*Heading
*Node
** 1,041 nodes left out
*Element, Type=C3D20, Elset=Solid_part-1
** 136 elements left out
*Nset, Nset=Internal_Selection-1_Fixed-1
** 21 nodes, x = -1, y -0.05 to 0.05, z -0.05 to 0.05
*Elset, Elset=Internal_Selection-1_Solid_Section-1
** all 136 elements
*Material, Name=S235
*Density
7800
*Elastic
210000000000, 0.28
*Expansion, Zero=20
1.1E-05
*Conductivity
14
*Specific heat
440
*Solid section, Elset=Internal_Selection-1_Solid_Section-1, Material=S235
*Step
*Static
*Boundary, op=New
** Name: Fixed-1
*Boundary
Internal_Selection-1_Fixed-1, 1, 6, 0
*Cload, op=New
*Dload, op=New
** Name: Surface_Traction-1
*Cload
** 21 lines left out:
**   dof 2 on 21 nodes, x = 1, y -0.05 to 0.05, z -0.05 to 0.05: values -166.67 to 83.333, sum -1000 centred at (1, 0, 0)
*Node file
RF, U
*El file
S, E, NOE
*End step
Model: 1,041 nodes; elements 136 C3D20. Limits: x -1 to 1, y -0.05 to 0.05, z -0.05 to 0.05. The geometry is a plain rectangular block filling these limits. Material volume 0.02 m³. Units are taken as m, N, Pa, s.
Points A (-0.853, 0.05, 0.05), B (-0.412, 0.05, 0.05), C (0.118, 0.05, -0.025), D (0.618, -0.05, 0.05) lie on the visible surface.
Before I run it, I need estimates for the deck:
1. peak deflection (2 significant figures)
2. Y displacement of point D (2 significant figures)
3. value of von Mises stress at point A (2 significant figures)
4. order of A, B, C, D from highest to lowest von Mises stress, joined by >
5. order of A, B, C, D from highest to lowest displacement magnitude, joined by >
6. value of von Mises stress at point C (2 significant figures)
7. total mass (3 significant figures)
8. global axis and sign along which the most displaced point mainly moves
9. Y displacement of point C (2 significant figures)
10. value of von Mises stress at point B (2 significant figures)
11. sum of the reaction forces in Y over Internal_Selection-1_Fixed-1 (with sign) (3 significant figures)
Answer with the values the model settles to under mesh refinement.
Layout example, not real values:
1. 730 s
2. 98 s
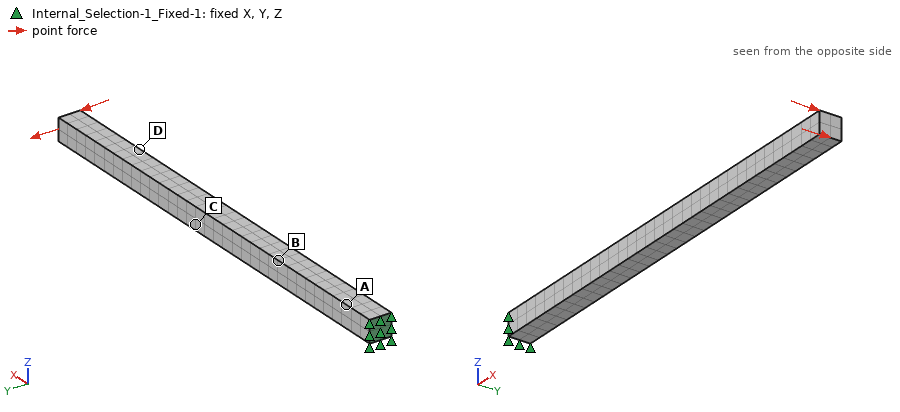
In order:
1. 0.0015 m
2. -0.0011 m
3. 1.1e+07 Pa
4. A > B > C > D
5. D > C > B > A
6. 5.3e+06 Pa
7. 156 kg
8. -Y
9. -5.8e-04 m
10. 8.5e+06 Pa
11. 1000 N
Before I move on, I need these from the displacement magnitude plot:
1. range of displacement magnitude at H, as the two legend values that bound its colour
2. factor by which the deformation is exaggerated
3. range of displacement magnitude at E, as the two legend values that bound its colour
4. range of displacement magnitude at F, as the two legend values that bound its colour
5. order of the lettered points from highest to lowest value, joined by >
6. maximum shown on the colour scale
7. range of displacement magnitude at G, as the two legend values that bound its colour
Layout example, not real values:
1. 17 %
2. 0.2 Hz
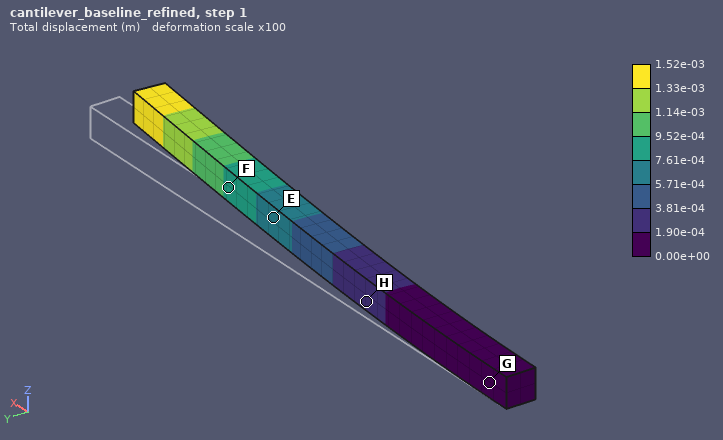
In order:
1. 1.90e-04 to 3.81e-04 m
2. 100
3. 5.71e-04 to 7.61e-04 m
4. 7.61e-04 to 9.52e-04 m
5. F > E > H > G
6. 1.52e-03 m
7. 0.00e+00 to 1.90e-04 m
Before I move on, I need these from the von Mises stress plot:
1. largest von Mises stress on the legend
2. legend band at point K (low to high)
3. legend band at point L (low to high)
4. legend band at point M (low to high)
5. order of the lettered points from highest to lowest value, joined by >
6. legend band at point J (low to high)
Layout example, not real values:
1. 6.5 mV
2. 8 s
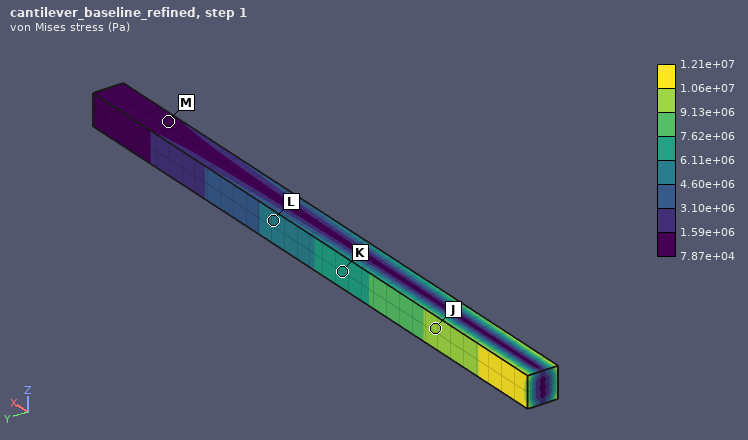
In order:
1. 1.21e+07 Pa
2. 6.11e+06 to 7.62e+06 Pa
3. 4.60e+06 to 6.11e+06 Pa
4. 7.87e+04 to 1.59e+06 Pa
5. J > K > L > M
6. 9.13e+06 to 1.06e+07 Pa
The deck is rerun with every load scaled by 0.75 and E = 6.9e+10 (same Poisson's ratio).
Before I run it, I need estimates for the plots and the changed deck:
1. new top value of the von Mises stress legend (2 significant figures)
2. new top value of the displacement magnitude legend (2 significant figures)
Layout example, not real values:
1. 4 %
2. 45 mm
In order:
1. 9.1e+06 Pa
2. 0.0035 m
